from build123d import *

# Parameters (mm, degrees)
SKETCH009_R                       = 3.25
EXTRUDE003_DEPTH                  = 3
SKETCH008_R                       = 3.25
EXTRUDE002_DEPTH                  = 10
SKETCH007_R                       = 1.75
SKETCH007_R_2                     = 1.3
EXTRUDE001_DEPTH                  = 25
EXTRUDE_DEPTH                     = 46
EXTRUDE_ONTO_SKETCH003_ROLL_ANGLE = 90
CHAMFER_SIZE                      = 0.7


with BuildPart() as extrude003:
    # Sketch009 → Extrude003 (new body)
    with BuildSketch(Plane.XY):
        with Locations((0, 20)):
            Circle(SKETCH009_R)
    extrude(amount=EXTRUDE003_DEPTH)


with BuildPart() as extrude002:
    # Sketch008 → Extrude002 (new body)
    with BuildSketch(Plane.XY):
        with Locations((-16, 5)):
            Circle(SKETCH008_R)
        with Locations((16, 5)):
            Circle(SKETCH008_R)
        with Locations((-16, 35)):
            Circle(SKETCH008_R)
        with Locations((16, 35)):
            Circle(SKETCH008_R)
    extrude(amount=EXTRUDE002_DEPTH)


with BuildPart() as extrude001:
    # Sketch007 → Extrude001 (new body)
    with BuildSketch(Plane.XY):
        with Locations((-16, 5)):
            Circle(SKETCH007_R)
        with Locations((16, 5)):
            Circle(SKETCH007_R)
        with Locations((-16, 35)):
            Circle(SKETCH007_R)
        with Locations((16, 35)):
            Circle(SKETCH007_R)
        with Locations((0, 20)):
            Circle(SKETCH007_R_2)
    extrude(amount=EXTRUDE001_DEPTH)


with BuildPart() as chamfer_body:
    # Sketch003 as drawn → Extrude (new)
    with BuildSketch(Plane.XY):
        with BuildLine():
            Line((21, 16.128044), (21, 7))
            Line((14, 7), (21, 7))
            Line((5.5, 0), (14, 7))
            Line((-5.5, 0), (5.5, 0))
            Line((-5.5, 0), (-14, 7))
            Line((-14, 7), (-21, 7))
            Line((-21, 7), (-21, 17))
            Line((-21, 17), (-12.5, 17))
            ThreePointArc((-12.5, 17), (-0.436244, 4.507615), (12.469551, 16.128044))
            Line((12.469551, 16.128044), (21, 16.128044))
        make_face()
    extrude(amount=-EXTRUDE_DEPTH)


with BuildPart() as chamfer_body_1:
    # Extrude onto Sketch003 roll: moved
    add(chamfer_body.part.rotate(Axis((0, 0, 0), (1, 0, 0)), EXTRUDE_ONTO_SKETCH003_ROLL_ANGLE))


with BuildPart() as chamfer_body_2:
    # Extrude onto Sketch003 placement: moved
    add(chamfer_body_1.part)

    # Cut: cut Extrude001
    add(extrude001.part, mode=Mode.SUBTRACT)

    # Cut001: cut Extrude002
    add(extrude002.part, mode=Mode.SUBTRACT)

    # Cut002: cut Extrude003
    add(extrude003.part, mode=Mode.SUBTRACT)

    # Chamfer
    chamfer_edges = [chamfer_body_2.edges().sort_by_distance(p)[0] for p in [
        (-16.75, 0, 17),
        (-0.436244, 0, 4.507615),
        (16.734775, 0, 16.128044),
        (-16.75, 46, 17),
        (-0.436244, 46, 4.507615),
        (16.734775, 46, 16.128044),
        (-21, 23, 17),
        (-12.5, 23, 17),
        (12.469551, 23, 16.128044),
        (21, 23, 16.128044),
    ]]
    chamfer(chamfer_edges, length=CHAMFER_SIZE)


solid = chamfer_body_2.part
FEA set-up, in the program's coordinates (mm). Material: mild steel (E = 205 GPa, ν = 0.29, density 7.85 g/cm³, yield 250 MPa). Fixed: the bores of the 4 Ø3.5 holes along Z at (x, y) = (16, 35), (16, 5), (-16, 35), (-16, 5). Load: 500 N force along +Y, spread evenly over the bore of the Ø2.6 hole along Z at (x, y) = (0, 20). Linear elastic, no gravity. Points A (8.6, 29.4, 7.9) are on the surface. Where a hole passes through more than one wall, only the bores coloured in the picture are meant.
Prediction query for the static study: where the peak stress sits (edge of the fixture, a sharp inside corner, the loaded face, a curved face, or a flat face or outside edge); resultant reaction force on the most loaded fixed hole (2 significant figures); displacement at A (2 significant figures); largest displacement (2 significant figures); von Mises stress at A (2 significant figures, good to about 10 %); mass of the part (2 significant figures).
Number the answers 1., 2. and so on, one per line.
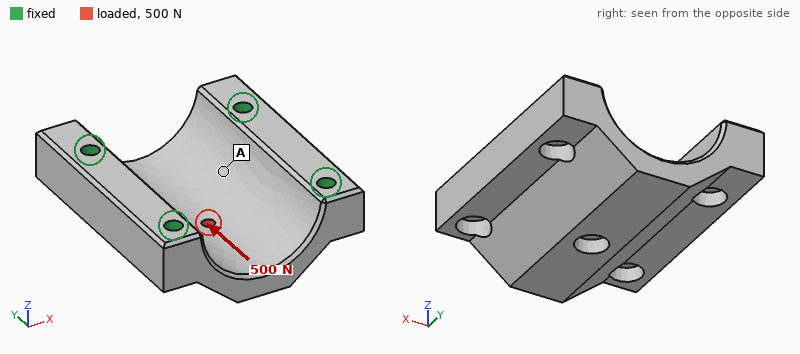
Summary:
1. the loaded face
2. 160 N
3. 0.20 µm
4. 0.97 µm
5. 3.2 MPa
6. 100 g
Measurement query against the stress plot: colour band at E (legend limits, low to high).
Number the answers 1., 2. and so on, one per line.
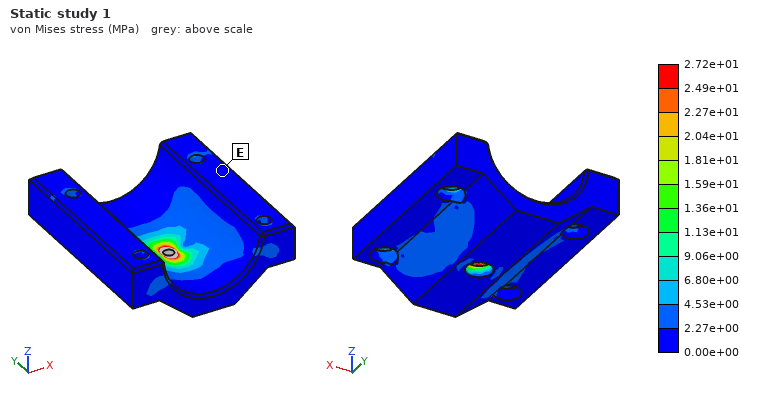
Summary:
1. 0.00e+00 to 2.27e+00 MPa
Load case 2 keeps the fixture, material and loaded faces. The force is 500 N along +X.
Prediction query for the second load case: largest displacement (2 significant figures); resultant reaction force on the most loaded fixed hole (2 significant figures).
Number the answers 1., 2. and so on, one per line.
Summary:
1. 1.2 µm
2. 140 N
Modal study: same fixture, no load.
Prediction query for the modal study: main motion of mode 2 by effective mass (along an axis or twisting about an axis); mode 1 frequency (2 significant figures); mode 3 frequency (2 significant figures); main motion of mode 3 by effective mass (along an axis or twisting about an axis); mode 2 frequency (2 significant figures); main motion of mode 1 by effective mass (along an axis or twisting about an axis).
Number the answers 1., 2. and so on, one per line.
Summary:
1. along Y
2. 24 kHz
3. 29 kHz
4. along Z
5. 26 kHz
6. along X
